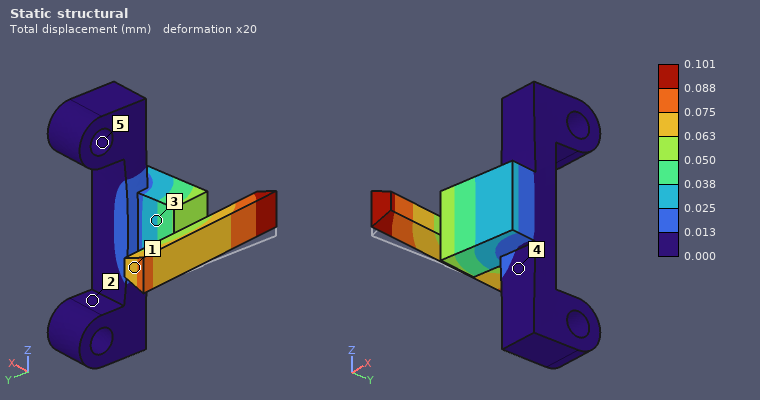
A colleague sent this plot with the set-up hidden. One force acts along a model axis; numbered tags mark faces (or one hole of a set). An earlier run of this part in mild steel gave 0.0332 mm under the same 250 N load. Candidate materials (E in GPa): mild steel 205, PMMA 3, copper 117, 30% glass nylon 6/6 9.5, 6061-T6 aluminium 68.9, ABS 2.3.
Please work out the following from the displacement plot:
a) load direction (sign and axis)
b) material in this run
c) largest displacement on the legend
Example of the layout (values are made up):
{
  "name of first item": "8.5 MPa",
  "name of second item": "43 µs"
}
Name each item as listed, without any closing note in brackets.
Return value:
{
  "load direction": "-Y",
  "material in this run": "6061-T6 aluminium",
  "largest displacement on the legend": "0.101 mm"
}
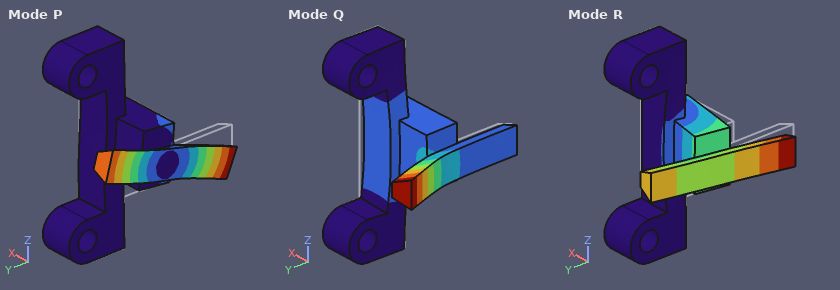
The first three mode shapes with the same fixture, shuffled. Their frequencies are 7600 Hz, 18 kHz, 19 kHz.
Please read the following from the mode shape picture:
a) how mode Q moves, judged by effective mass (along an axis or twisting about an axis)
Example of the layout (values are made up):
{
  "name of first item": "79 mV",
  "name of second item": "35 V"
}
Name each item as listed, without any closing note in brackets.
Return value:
{
  "how mode Q moves, judged by effective mass": "along X"
}
